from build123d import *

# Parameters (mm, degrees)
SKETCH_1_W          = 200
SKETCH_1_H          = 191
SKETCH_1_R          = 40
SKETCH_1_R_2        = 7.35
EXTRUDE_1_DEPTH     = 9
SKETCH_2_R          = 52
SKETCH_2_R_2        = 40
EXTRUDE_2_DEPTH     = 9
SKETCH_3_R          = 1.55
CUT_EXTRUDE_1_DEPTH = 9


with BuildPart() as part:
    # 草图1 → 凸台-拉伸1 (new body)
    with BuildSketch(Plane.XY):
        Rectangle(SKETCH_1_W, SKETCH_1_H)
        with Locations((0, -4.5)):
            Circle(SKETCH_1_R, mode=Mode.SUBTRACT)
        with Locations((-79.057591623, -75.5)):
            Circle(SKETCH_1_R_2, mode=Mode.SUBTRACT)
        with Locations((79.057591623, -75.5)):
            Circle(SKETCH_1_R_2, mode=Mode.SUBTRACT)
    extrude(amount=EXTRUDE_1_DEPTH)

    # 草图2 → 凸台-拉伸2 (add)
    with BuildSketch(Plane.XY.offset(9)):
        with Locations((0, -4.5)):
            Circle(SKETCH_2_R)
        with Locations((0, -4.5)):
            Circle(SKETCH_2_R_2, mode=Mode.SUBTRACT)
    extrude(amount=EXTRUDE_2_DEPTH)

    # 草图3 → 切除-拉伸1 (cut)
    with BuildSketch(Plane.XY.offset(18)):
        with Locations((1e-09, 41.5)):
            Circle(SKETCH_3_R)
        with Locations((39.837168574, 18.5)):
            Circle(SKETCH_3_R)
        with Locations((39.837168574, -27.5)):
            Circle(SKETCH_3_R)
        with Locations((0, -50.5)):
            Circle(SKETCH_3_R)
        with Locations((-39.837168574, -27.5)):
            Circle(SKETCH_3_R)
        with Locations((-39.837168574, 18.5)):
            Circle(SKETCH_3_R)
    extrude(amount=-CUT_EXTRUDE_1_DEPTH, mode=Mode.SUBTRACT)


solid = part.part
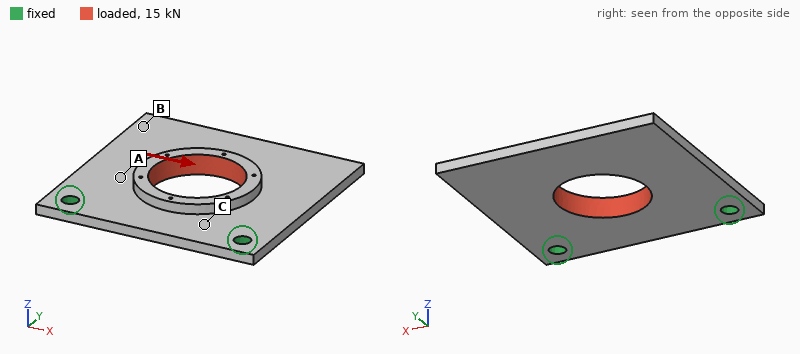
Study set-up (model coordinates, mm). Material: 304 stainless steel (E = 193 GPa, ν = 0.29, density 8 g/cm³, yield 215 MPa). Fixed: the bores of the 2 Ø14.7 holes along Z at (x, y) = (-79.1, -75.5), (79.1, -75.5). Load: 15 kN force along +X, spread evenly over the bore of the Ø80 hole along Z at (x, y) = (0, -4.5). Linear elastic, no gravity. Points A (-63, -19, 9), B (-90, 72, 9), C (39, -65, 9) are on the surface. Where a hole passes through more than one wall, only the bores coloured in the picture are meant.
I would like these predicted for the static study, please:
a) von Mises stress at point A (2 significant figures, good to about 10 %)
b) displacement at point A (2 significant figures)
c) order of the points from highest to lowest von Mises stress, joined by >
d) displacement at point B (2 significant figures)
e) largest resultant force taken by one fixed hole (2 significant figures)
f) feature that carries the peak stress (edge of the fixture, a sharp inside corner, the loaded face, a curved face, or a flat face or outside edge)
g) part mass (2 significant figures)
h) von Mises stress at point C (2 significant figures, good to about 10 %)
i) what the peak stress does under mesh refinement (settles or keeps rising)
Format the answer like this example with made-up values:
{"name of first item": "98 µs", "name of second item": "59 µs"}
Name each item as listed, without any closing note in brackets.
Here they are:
{"von Mises stress at point A": "27 MPa", "displacement at point A": "16 µm", "order of the points from highest to lowest von Mises stress, joined by >": "A > C > B", "displacement at point B": "38 µm", "largest resultant force taken by one fixed hole": "9.7 kN", "feature that carries the peak stress": "edge of the fixture", "part mass": "2.6 kg", "von Mises stress at point C": "19 MPa", "what the peak stress does under mesh refinement": "keeps rising"}
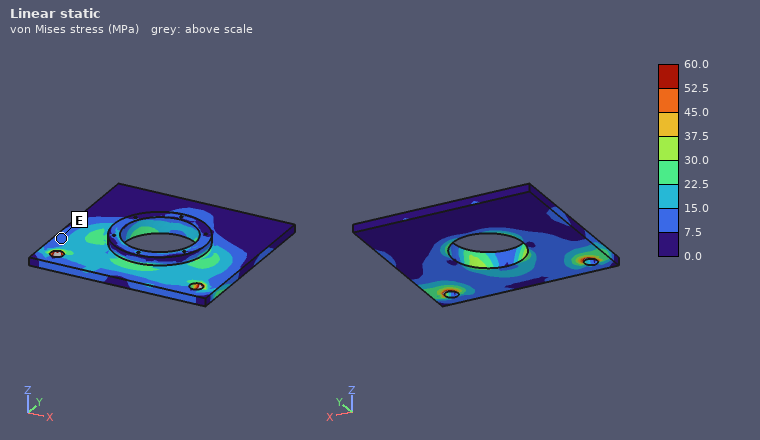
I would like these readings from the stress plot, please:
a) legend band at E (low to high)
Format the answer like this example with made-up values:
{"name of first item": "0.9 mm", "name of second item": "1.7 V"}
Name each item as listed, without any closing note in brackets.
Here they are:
{"legend band at E": "7.5 to 15.0 MPa"}
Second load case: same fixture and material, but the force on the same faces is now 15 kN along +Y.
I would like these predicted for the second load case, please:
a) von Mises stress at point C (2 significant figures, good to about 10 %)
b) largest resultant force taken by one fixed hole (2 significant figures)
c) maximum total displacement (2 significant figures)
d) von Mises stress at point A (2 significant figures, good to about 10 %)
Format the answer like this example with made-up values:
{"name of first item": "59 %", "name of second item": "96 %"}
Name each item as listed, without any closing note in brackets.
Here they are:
{"von Mises stress at point C": "27 MPa", "largest resultant force taken by one fixed hole": "7.8 kN", "maximum total displacement": "0.29 mm", "von Mises stress at point A": "23 MPa"}
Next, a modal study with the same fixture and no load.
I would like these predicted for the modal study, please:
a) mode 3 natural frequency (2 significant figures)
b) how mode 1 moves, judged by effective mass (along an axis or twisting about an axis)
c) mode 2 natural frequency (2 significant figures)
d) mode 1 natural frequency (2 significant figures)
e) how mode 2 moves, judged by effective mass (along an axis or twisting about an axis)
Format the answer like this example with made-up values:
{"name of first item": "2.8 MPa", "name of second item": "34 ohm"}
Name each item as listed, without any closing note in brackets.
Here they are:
{"mode 3 natural frequency": "1600 Hz", "how mode 1 moves, judged by effective mass": "along Z", "mode 2 natural frequency": "590 Hz", "mode 1 natural frequency": "230 Hz", "how mode 2 moves, judged by effective mass": "twisting about Y"}
